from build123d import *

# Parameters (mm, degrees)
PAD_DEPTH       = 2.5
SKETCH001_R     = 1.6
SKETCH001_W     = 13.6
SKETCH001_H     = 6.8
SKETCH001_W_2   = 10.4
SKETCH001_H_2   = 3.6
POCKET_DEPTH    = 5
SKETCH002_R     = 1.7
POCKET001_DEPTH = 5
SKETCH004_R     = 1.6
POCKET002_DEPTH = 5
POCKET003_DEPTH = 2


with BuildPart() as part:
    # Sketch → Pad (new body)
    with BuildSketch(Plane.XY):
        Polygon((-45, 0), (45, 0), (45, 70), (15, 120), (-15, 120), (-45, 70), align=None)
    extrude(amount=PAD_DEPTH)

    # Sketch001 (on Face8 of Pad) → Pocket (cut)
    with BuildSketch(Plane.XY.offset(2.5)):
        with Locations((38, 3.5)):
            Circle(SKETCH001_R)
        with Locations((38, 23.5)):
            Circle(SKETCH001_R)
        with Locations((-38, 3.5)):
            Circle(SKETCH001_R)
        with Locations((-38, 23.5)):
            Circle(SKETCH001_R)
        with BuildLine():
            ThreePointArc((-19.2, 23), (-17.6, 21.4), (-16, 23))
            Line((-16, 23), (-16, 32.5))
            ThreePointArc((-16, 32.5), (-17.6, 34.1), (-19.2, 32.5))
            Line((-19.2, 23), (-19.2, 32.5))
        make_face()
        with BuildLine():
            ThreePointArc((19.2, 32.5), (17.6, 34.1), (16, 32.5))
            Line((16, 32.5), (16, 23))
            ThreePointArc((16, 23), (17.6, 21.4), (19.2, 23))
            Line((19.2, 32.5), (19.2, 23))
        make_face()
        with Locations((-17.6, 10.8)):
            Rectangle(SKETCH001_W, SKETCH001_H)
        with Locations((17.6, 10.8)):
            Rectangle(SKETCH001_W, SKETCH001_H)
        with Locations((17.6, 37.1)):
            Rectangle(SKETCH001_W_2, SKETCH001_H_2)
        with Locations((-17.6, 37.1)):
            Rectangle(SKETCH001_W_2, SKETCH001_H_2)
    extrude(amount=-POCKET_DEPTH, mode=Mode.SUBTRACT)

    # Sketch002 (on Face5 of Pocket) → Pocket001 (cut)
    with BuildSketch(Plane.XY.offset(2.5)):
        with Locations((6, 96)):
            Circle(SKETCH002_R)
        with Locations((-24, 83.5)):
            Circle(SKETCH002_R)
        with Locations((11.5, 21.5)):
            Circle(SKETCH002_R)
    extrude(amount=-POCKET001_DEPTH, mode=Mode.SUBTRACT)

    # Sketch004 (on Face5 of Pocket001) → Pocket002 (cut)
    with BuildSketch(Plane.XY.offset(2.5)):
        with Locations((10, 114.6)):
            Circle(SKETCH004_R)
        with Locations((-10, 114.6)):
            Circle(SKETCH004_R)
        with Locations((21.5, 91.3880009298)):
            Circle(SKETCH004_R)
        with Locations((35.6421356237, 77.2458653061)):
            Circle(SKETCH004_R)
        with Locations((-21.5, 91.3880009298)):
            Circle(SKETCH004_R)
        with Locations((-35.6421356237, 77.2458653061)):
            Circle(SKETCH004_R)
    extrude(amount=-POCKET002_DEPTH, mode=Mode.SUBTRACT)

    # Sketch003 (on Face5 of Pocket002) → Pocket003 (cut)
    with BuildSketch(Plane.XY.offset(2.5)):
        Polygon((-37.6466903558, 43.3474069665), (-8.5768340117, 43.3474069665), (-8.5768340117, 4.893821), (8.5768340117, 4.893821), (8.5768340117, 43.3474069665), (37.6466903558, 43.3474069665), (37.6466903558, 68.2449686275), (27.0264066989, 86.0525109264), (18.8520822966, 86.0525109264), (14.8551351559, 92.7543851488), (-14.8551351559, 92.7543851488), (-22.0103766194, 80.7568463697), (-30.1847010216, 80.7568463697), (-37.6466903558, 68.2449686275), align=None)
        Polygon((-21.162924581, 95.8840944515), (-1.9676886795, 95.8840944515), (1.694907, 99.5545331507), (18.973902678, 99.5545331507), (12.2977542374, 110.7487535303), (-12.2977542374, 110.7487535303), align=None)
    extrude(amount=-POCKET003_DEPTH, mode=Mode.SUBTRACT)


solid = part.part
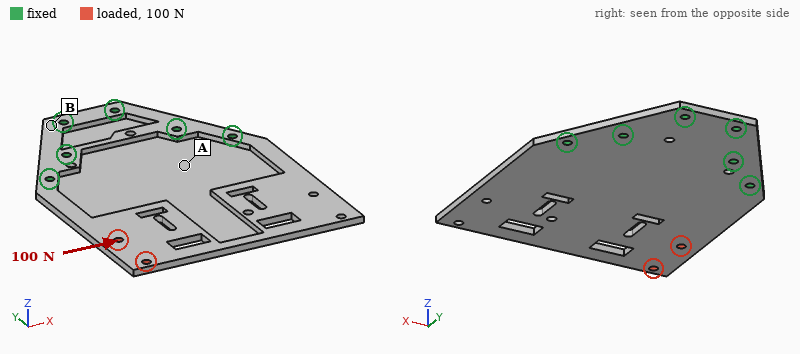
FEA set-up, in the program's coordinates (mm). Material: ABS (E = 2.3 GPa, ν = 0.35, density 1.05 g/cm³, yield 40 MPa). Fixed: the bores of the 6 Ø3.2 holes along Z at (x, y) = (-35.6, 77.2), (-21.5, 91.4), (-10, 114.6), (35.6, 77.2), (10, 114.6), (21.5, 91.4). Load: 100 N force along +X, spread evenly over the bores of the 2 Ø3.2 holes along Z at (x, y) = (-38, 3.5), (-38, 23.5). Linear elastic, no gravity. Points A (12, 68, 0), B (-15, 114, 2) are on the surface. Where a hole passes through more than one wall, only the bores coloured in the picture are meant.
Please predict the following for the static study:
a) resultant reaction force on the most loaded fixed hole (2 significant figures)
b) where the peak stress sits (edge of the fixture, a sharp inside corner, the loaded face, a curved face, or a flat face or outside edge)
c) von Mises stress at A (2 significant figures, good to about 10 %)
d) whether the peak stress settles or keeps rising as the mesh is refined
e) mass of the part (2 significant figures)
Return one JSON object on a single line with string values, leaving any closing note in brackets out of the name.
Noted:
{"resultant reaction force on the most loaded fixed hole": "90 N", "where the peak stress sits": "edge of the fixture", "von Mises stress at A": "4.2 MPa", "whether the peak stress settles or keeps rising as the mesh is refined": "keeps rising", "mass of the part": "14 g"}
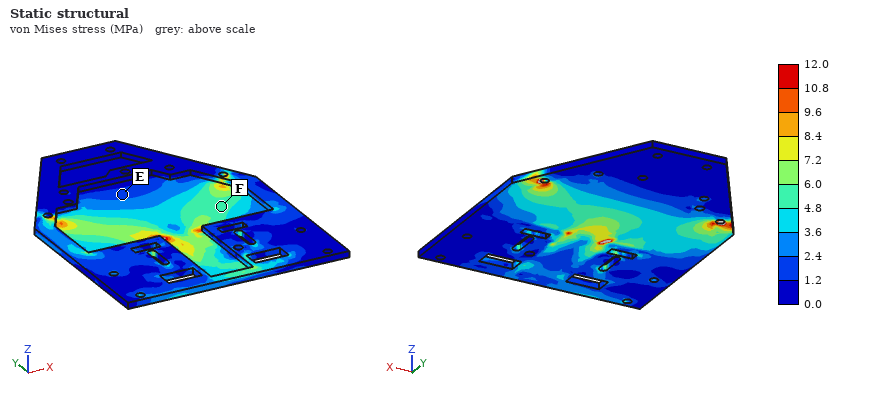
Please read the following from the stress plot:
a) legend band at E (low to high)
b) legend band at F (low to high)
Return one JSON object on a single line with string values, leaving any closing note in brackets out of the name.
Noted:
{"legend band at E": "1.2 to 2.4 MPa", "legend band at F": "4.8 to 6.0 MPa"}
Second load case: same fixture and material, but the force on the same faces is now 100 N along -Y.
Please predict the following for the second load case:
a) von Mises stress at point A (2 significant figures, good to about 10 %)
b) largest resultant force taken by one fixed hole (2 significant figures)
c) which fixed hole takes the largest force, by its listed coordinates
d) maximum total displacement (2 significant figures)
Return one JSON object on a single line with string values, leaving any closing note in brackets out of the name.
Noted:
{"von Mises stress at point A": "0.56 MPa", "largest resultant force taken by one fixed hole": "89 N", "which fixed hole takes the largest force, by its listed coordinates": "(-35.6, 77.2)", "maximum total displacement": "1.7 mm"}
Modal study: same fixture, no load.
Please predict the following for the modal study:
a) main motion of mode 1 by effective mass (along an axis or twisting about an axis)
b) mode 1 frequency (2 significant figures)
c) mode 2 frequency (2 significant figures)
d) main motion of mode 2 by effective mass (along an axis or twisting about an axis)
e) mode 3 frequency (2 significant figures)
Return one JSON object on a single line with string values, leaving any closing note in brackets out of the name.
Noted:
{"main motion of mode 1 by effective mass": "along Z", "mode 1 frequency": "58 Hz", "mode 2 frequency": "140 Hz", "main motion of mode 2 by effective mass": "twisting about Y", "mode 3 frequency": "280 Hz"}
